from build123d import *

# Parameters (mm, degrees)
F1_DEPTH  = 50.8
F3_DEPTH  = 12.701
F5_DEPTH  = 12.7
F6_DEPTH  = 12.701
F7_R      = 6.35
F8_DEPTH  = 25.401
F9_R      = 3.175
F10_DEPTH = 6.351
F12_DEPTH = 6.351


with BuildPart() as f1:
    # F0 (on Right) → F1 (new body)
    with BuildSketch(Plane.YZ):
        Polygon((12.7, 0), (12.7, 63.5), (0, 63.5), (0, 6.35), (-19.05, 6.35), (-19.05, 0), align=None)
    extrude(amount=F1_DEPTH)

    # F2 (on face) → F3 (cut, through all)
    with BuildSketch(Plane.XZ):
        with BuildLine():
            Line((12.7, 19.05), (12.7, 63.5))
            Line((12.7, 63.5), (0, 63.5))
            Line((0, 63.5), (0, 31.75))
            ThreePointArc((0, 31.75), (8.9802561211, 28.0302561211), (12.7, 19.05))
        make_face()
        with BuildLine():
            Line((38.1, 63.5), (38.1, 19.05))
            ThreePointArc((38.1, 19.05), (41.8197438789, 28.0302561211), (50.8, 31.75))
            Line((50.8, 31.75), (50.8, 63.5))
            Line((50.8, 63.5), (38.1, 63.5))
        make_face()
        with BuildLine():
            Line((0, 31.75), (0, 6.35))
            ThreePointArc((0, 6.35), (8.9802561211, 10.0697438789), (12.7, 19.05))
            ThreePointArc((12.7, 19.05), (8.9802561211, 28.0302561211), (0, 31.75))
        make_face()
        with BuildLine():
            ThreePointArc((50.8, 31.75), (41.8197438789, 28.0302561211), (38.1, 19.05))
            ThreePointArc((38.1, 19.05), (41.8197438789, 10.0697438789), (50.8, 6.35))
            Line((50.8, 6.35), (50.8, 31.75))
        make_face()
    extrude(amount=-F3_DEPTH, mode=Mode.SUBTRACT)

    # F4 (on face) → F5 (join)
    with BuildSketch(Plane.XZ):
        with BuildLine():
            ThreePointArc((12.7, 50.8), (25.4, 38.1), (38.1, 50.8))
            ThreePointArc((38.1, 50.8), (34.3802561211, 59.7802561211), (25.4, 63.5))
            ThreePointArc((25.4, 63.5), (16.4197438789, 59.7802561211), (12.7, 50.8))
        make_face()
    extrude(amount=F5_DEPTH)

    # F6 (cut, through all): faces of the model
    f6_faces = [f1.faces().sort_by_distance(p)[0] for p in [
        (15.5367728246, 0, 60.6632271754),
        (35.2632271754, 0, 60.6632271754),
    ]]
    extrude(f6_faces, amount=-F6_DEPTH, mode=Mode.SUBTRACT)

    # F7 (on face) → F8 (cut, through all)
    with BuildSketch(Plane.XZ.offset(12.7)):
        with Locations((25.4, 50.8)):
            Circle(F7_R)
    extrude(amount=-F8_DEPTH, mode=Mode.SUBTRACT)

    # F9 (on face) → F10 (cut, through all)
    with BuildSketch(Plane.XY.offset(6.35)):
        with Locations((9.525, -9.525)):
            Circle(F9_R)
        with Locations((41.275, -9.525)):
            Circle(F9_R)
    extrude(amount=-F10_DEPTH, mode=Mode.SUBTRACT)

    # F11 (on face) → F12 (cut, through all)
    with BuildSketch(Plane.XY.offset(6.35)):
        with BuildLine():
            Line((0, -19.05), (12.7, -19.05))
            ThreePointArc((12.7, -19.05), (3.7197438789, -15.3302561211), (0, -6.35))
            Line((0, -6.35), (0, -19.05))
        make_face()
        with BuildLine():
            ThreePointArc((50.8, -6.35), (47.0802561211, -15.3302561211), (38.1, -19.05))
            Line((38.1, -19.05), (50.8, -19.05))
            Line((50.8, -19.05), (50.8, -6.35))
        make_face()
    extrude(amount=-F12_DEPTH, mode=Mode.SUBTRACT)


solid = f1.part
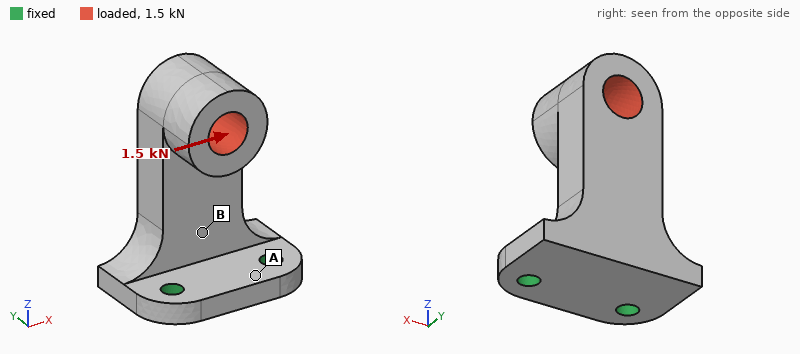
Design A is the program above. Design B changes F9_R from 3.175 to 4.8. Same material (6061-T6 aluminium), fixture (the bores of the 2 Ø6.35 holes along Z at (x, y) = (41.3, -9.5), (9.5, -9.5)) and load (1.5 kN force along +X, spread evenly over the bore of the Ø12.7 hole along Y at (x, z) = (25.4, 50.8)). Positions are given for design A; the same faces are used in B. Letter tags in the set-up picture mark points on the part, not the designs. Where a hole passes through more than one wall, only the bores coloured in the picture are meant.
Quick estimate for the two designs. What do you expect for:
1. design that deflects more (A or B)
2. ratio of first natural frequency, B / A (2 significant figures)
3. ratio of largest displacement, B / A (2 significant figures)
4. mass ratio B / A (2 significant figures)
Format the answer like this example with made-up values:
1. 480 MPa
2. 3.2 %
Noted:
1. A
2. 1.1
3. 0.85
4. 0.98
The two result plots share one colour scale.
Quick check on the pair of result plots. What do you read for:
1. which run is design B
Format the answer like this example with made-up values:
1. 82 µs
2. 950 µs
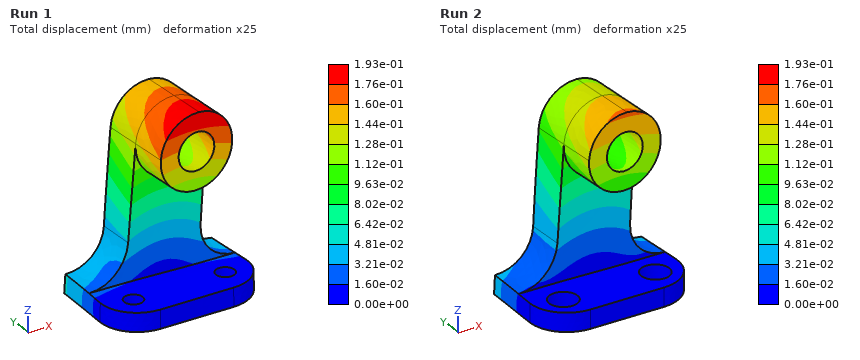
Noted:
1. Run 2
